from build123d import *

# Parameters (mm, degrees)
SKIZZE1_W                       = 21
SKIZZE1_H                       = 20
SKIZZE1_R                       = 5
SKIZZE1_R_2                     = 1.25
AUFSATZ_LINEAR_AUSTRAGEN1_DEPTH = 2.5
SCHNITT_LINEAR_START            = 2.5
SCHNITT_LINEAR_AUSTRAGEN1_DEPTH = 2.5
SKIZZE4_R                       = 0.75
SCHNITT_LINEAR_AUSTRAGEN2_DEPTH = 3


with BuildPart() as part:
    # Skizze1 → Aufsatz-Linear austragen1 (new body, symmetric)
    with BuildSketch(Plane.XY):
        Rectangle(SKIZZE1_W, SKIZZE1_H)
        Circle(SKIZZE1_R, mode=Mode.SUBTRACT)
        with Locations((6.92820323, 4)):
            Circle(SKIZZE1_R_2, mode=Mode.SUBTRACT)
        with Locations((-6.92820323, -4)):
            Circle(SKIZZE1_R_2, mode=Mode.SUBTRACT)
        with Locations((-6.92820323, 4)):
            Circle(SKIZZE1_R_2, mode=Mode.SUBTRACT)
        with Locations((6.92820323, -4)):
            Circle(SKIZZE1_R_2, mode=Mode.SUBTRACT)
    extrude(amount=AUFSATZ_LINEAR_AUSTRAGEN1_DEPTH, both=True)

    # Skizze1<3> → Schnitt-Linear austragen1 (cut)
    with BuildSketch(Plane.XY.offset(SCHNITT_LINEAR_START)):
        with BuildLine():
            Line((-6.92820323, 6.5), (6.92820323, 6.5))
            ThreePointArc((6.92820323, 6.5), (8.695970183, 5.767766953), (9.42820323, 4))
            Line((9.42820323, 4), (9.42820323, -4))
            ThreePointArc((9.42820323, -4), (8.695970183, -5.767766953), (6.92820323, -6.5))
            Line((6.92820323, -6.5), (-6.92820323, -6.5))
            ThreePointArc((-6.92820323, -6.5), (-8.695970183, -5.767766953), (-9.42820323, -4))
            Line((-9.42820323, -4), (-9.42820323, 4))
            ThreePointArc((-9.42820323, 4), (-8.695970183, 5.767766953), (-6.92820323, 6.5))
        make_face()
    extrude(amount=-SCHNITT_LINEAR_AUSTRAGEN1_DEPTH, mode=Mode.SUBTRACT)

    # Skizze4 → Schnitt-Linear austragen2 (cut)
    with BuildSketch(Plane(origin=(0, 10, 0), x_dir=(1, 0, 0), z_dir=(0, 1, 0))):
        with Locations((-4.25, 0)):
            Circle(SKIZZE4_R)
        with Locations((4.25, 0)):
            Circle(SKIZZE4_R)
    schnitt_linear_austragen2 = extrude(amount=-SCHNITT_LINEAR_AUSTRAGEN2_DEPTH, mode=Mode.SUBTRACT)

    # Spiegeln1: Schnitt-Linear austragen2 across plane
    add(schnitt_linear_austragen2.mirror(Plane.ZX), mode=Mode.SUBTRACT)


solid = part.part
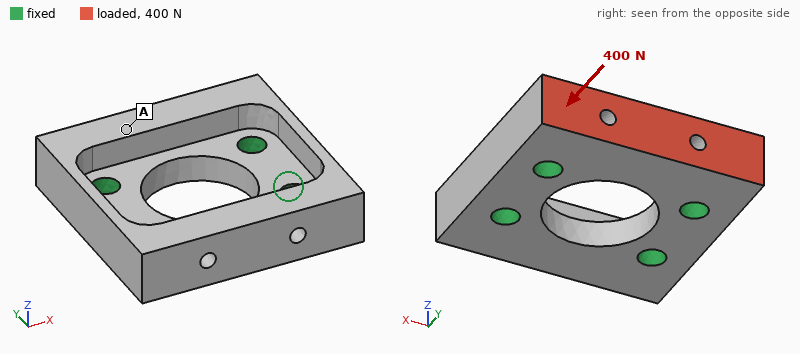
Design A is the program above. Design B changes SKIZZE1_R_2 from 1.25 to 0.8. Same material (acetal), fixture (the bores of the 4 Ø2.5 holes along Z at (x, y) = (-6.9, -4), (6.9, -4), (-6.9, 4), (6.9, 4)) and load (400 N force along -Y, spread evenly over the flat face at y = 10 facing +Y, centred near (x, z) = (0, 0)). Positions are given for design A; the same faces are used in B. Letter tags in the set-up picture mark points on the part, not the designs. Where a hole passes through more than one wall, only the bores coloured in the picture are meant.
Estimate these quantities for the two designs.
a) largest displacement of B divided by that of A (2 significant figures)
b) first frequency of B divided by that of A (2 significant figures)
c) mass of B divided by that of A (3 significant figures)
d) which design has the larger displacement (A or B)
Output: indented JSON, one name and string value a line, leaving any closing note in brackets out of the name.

{
  "largest displacement of B divided by that of A": "1.2",
  "first frequency of B divided by that of A": "0.86",
  "mass of B divided by that of A": "1.02",
  "which design has the larger displacement": "B"
}
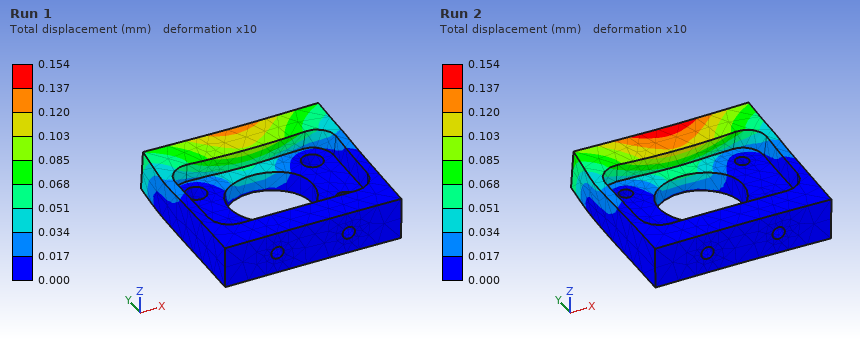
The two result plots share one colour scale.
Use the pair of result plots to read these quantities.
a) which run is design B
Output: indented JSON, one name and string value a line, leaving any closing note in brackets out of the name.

{
  "which run is design B": "Run 2"
}
